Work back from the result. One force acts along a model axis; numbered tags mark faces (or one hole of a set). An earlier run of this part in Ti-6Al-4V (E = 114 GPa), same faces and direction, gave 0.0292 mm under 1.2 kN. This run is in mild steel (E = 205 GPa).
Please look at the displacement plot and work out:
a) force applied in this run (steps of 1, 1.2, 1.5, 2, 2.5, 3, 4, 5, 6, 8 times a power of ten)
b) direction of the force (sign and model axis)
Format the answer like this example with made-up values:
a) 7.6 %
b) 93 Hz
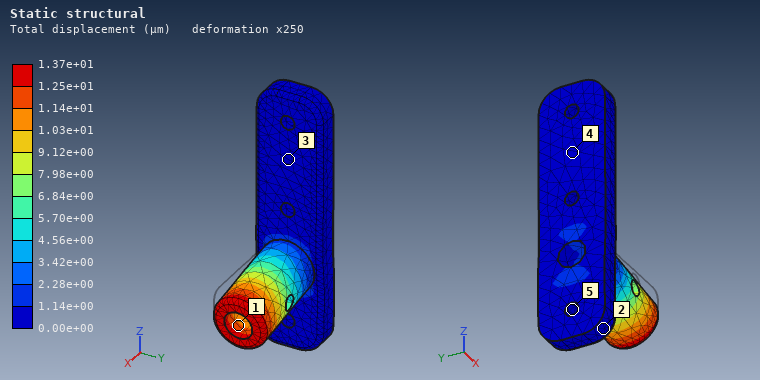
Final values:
a) 1 kN
b) -Z
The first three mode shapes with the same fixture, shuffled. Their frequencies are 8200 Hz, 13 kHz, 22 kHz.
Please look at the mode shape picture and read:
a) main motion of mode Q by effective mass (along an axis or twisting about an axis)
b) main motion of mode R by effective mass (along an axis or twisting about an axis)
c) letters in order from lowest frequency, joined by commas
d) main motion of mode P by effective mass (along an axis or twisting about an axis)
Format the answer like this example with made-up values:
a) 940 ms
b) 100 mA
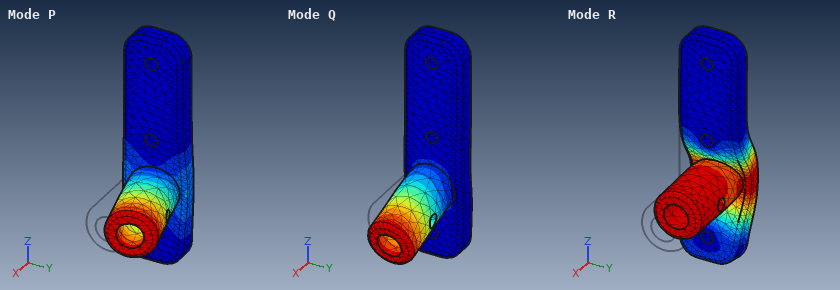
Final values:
a) along Z
b) along X
c) P, Q, R
d) along Y
